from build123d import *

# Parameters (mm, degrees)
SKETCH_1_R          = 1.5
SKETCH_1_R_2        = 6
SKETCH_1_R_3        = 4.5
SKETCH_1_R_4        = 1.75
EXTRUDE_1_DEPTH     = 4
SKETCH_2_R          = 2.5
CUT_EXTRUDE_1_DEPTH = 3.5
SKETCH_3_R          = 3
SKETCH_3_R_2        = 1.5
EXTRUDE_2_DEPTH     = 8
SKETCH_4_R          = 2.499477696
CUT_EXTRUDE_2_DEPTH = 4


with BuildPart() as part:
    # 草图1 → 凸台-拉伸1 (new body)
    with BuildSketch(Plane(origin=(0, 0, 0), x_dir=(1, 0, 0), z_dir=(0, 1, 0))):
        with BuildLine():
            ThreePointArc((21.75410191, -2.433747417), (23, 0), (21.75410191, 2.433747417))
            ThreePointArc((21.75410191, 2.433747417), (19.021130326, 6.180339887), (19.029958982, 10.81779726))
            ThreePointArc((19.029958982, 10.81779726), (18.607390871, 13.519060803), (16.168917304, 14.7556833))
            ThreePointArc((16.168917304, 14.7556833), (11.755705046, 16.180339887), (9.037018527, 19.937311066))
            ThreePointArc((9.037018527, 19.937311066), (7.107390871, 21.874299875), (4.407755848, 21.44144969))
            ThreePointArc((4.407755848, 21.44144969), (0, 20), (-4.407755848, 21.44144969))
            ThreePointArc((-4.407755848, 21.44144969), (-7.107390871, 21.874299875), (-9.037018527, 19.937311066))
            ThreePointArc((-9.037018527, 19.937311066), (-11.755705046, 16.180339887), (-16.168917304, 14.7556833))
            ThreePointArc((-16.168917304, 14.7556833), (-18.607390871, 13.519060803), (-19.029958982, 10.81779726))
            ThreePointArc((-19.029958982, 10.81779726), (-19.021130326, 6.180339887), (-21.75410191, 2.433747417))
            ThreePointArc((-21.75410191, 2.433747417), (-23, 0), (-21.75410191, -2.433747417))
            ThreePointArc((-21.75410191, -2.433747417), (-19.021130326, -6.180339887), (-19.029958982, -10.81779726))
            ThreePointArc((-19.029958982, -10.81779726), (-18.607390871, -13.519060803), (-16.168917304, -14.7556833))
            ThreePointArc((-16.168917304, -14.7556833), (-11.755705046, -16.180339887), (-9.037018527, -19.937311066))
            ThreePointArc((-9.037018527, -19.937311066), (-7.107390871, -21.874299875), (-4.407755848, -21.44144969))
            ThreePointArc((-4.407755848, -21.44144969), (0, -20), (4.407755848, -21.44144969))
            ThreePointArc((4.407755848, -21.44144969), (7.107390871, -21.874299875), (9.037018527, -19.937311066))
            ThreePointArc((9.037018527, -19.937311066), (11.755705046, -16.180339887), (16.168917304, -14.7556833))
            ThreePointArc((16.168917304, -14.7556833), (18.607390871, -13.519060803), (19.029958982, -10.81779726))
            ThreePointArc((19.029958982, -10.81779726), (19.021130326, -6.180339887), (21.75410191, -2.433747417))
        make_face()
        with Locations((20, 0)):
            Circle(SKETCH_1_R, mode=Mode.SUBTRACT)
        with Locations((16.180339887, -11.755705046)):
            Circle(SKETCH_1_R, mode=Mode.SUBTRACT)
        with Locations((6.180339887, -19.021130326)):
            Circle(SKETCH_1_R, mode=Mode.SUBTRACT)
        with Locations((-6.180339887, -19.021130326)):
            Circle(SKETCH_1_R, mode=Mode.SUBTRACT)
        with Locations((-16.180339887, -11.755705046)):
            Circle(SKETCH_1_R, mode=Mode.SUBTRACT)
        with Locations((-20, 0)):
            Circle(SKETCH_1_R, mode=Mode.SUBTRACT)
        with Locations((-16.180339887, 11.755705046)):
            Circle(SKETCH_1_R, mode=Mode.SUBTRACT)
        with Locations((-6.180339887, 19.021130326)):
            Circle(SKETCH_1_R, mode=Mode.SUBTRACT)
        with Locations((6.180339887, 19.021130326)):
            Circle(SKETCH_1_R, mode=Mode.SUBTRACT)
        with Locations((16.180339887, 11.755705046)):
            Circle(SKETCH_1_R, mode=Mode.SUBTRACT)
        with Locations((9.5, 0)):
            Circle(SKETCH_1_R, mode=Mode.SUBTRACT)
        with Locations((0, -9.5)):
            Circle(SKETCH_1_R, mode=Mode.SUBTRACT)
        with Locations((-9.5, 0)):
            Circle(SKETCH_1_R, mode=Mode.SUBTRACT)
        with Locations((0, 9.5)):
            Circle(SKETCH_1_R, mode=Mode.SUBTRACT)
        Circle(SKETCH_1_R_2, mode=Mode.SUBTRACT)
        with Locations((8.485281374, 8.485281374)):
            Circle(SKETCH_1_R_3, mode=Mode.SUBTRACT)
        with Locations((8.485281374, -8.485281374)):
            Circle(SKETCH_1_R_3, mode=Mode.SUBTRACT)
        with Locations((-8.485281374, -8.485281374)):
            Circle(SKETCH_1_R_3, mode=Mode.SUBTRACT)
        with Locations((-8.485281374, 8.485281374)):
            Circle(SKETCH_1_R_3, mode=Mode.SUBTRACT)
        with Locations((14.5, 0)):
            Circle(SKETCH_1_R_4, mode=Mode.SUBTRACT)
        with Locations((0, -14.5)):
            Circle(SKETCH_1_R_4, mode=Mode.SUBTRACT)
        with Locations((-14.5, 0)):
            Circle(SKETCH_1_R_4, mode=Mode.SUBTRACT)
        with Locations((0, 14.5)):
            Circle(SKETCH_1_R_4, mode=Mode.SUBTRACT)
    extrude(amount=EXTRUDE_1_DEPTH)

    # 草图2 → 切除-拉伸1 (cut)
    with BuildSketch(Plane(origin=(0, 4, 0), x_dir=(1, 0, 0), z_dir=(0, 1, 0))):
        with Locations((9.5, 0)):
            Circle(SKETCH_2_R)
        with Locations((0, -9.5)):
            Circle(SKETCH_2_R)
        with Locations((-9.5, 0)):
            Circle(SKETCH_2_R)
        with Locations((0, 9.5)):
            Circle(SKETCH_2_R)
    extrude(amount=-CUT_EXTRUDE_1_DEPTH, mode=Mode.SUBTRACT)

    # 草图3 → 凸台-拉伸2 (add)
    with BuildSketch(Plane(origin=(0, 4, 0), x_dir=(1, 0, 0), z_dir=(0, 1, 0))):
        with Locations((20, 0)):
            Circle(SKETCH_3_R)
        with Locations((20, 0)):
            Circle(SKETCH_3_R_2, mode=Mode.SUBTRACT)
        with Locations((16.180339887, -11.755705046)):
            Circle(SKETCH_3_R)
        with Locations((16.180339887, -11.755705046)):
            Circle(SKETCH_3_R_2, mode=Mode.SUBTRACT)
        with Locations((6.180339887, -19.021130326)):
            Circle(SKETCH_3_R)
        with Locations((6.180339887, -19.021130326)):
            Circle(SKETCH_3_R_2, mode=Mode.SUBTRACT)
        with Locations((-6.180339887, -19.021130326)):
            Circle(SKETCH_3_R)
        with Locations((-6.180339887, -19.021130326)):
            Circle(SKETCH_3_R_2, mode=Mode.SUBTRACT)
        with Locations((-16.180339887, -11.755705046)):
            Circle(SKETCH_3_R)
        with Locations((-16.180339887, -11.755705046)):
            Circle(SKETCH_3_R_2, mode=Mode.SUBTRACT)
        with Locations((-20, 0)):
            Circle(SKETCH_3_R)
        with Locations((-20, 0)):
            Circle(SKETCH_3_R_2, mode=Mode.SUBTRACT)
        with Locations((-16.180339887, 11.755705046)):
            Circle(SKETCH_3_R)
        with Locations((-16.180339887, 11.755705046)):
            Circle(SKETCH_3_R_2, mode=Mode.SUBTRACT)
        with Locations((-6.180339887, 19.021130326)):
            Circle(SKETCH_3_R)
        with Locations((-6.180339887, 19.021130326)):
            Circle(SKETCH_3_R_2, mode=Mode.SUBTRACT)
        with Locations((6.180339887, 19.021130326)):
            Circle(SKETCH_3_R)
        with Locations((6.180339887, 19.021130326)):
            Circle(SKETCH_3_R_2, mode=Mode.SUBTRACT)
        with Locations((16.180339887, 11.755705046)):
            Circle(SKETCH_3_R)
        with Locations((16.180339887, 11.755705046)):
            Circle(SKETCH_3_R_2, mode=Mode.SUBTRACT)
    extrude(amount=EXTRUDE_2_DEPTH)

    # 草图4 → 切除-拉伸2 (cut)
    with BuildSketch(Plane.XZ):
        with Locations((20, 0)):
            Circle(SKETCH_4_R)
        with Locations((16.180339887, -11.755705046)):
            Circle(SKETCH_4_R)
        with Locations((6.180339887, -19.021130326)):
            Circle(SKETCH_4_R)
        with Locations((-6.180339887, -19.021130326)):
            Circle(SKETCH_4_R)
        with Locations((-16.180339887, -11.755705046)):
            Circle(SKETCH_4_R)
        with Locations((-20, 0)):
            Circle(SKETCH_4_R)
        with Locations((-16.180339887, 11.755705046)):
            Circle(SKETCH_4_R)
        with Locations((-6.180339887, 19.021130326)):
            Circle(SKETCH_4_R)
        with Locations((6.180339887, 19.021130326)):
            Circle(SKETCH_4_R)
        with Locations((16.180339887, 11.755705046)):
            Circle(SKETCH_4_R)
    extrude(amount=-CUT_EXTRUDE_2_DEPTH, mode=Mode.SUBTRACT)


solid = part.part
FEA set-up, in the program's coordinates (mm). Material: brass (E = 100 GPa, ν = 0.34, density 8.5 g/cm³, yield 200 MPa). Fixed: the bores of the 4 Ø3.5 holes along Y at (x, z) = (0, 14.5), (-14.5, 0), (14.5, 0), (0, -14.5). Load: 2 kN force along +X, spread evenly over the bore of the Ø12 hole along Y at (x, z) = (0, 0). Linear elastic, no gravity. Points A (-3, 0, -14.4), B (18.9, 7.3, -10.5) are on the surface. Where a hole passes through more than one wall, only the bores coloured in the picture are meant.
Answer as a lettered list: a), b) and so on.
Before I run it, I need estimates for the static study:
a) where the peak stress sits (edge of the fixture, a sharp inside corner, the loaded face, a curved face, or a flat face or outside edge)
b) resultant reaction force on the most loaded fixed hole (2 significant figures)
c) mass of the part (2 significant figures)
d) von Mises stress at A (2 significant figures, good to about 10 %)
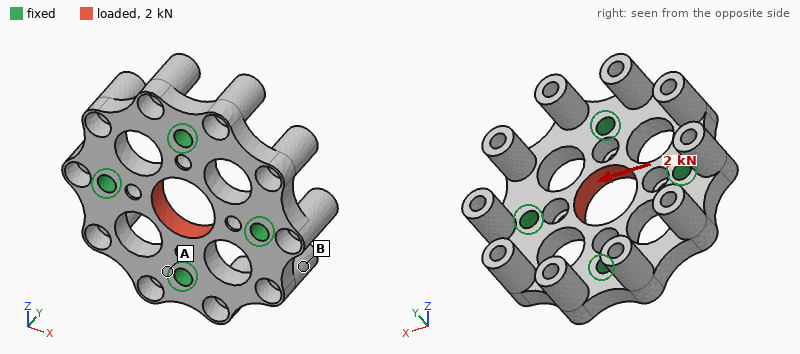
a) a curved face
b) 710 N
c) 40 g
d) 14 MPa
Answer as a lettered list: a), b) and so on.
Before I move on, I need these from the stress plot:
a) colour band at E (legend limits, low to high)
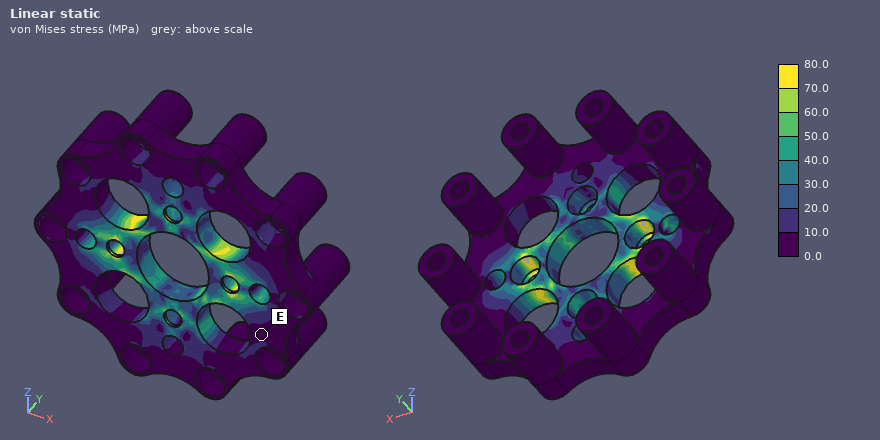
a) 0.0 to 10.0 MPa
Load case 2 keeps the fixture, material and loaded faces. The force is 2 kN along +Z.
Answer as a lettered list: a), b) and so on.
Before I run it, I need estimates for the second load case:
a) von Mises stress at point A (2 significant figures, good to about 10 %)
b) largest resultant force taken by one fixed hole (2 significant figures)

a) 24 MPa
b) 720 N
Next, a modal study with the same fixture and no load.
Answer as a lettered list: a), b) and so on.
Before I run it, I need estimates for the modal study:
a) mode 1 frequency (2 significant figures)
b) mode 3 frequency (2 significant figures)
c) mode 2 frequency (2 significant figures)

a) 8700 Hz
b) 8900 Hz
c) 8800 Hz
